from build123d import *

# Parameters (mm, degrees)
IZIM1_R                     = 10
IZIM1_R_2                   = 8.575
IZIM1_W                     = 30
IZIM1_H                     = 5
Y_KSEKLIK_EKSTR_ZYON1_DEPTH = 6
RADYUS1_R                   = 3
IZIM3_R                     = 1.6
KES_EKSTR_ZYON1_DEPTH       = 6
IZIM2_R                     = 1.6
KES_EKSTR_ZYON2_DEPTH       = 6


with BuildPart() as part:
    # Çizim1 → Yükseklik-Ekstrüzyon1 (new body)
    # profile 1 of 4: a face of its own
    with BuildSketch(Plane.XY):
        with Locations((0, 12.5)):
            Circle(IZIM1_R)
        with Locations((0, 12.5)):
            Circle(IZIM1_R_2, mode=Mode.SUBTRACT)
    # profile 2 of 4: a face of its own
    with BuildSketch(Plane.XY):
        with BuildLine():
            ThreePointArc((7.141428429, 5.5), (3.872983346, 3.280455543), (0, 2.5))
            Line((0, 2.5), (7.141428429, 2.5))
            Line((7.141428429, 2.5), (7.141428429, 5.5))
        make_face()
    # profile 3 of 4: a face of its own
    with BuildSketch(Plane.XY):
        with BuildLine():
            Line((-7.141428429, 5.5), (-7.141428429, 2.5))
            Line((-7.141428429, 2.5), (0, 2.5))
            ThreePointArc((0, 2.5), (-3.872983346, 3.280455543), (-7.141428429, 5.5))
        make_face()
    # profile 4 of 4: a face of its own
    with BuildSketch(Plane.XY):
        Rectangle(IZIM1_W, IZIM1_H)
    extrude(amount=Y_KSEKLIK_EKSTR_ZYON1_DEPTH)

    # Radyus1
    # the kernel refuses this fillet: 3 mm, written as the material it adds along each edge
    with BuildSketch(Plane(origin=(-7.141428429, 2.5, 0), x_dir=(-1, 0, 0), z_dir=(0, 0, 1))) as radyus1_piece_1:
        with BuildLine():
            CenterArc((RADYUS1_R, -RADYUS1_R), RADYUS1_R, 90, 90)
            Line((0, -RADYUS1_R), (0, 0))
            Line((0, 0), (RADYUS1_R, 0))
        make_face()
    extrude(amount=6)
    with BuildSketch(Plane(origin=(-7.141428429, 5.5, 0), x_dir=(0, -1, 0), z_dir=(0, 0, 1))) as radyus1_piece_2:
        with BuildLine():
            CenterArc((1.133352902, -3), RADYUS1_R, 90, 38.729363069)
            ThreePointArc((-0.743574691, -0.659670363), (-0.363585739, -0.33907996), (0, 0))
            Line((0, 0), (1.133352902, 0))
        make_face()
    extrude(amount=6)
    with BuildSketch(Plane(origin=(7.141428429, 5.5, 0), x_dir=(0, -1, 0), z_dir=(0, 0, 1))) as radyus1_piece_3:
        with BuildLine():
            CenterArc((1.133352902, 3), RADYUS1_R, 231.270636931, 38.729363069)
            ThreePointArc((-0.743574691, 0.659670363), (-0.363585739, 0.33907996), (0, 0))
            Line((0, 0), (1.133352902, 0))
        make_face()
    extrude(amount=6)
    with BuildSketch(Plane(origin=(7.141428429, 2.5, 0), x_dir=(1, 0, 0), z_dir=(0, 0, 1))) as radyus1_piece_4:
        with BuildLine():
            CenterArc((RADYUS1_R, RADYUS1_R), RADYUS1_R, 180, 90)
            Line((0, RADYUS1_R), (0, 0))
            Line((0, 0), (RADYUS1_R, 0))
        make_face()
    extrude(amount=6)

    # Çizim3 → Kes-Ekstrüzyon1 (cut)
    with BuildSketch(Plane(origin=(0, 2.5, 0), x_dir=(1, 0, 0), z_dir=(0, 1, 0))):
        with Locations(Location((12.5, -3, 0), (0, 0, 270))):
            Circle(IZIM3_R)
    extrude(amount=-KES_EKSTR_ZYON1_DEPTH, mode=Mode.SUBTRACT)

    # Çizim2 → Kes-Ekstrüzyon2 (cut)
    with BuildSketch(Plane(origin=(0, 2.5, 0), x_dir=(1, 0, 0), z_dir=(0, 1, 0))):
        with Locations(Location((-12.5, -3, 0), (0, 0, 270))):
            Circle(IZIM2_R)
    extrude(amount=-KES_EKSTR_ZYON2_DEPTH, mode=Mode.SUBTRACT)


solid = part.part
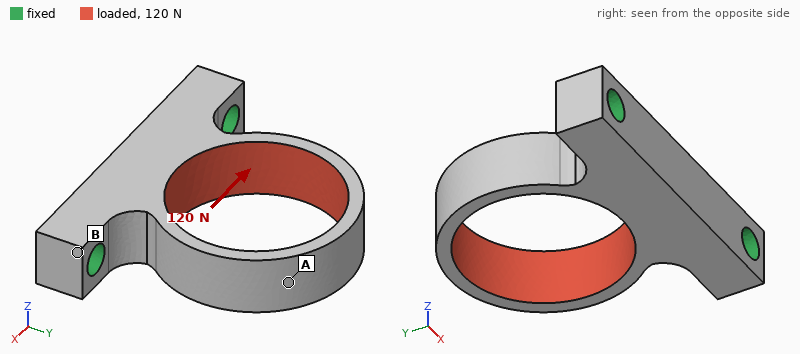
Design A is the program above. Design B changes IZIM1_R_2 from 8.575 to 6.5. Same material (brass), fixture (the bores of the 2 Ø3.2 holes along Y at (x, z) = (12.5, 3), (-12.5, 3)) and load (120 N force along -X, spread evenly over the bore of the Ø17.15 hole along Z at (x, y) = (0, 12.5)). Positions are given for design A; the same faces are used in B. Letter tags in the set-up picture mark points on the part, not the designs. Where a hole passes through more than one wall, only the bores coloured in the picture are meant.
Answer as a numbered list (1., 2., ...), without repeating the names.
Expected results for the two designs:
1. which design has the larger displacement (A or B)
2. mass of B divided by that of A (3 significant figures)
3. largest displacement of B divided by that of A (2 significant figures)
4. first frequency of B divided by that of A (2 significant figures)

1. A
2. 1.41
3. 0.092
4. 1.2
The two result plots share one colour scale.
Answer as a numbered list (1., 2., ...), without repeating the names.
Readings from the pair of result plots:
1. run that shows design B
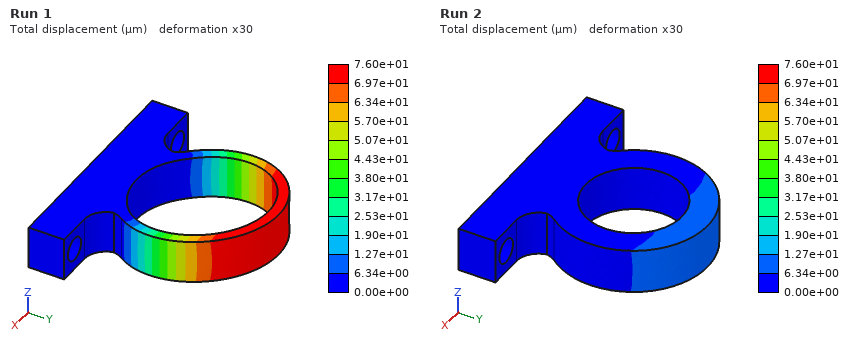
1. Run 2
